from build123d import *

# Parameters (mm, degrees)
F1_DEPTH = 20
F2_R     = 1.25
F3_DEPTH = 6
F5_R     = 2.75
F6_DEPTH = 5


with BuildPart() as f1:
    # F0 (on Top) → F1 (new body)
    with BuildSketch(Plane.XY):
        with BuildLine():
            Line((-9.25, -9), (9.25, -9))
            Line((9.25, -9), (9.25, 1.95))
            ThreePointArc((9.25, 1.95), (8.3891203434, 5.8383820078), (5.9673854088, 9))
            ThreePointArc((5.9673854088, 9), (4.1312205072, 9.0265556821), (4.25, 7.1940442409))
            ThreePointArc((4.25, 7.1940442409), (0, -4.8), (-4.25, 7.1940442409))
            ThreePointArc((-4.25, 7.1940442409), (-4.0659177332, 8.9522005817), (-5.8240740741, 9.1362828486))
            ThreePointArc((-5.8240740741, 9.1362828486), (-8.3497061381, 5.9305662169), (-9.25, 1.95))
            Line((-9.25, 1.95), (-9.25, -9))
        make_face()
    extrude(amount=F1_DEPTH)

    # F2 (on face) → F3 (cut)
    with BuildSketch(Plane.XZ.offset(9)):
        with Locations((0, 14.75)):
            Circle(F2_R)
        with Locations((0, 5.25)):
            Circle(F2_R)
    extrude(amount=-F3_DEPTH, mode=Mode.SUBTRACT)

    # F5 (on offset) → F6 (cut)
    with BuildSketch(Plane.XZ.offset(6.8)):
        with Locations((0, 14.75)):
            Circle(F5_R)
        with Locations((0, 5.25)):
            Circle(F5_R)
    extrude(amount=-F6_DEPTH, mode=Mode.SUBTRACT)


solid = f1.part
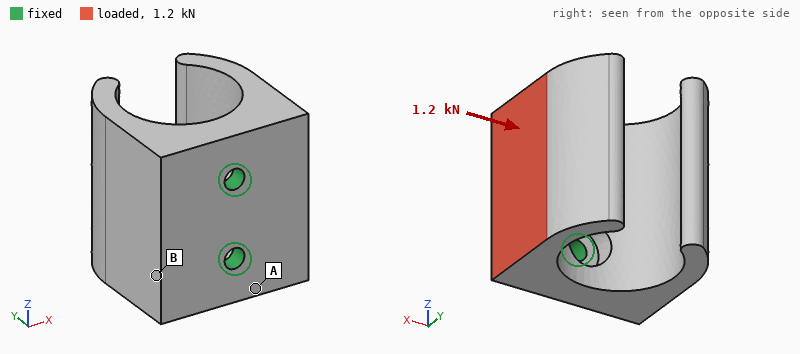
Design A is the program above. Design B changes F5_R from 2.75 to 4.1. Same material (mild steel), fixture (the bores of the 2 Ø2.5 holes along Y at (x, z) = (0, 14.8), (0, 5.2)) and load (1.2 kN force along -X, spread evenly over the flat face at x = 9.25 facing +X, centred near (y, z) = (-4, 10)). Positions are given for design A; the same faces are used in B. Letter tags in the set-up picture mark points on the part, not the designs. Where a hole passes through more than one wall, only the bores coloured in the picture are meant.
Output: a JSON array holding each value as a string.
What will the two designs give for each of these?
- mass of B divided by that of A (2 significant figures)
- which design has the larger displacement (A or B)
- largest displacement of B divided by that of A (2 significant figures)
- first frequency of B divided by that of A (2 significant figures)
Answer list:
["0.96", "B", "1.3", "0.92"]
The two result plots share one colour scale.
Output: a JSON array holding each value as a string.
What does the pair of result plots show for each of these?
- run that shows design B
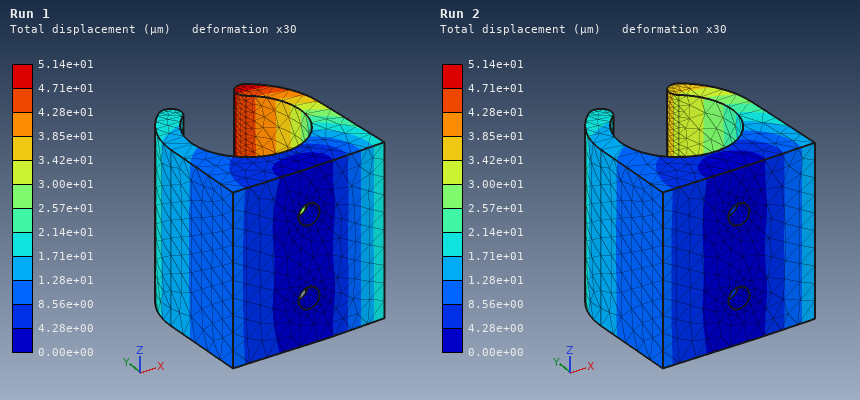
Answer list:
["Run 1"]
